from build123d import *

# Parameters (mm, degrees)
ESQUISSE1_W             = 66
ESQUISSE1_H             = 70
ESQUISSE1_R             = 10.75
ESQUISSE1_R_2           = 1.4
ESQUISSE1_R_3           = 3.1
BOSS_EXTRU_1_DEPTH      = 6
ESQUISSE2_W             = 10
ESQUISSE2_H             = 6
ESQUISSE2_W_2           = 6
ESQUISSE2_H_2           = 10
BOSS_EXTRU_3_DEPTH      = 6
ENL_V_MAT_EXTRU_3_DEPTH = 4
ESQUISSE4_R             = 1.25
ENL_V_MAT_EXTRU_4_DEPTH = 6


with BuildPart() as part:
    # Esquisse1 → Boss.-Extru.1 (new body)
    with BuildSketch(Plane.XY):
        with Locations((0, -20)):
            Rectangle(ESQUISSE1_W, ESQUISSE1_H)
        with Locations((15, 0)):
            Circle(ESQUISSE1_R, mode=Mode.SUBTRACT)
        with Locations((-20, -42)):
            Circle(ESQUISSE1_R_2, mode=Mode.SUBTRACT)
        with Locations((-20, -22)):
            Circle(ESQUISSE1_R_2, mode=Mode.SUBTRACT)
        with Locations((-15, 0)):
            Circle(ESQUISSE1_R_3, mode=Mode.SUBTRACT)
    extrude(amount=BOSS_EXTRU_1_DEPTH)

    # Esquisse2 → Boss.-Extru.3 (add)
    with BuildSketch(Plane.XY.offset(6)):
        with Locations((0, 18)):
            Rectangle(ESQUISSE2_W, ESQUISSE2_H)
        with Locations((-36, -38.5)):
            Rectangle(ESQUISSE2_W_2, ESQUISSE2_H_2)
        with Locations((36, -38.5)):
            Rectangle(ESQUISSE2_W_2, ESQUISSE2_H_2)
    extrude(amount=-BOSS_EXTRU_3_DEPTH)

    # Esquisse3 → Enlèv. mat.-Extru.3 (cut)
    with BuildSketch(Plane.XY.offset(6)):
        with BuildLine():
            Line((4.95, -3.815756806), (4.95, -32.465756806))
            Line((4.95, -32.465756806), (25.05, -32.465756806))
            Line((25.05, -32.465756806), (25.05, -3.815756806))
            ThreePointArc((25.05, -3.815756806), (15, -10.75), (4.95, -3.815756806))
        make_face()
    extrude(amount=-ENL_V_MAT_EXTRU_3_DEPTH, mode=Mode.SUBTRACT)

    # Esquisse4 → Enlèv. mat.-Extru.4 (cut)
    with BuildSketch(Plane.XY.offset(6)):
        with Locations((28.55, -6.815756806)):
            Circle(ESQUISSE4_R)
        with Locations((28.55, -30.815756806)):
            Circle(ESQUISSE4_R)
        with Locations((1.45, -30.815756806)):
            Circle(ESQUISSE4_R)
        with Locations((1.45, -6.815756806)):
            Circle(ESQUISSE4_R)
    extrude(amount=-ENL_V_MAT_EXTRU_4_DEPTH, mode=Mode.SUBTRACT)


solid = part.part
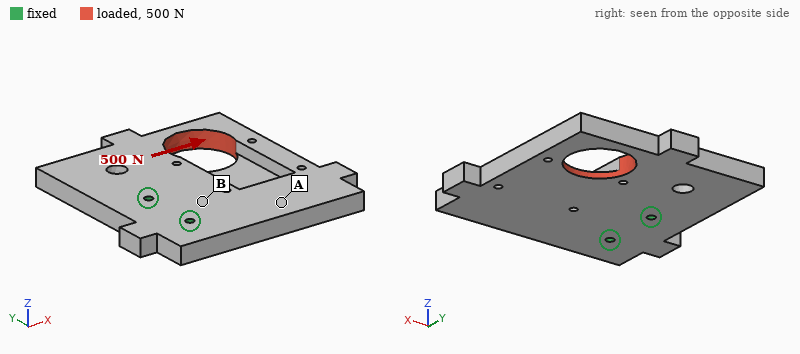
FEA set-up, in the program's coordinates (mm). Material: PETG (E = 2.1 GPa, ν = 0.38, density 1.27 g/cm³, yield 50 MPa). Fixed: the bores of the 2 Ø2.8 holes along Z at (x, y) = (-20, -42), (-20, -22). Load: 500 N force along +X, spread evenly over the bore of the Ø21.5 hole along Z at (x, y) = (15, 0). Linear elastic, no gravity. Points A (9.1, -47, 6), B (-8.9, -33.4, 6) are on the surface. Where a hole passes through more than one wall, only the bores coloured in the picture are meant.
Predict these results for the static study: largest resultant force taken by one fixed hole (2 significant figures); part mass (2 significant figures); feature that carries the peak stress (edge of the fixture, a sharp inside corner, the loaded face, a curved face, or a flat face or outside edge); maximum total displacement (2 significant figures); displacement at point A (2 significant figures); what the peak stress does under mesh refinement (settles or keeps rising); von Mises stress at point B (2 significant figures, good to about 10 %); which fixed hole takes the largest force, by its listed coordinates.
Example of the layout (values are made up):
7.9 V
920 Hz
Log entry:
1.1 kN
31 g
edge of the fixture
0.65 mm
0.20 mm
keeps rising
5.6 MPa
(-20, -22)
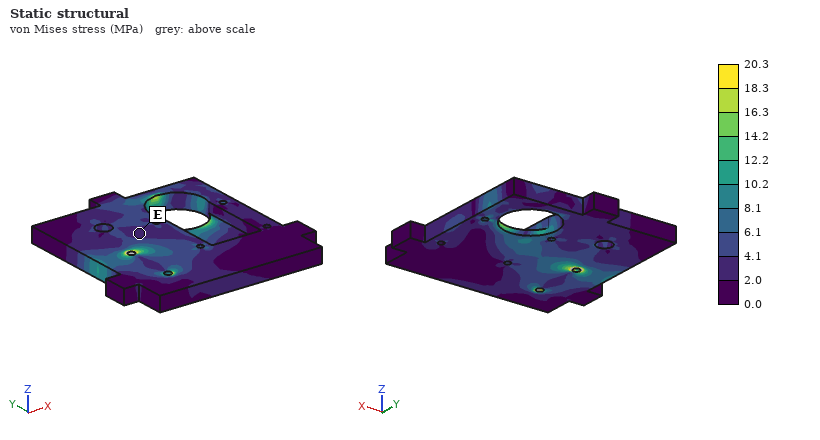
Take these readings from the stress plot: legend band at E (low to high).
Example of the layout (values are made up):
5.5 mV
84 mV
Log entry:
2.0 to 4.1 MPa
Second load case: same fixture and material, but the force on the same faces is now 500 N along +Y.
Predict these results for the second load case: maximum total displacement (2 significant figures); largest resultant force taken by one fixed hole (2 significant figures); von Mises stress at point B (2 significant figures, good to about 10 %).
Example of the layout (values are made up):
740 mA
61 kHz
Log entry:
0.65 mm
860 N
7.6 MPa
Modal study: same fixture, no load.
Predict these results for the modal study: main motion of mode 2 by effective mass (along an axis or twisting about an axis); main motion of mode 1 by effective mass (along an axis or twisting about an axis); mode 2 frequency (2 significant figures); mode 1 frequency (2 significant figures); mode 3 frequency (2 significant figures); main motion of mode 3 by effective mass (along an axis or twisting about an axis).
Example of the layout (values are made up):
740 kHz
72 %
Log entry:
twisting about X
along Z
540 Hz
360 Hz
950 Hz
along Z
